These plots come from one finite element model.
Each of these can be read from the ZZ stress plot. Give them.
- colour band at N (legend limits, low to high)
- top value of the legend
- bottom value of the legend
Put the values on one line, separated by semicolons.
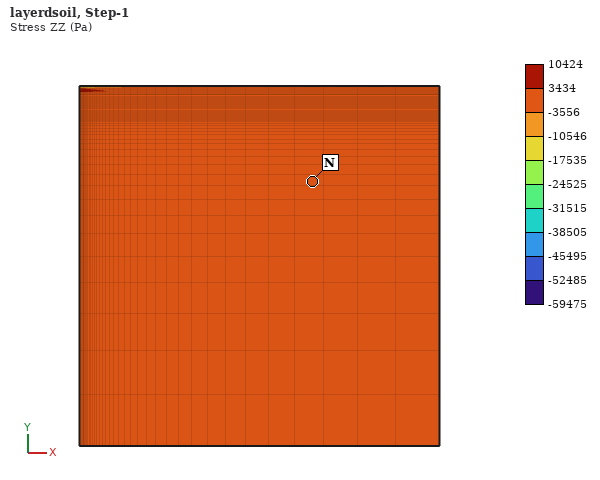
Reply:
-3556 to 3434 Pa; 10424 Pa; -59475 Pa
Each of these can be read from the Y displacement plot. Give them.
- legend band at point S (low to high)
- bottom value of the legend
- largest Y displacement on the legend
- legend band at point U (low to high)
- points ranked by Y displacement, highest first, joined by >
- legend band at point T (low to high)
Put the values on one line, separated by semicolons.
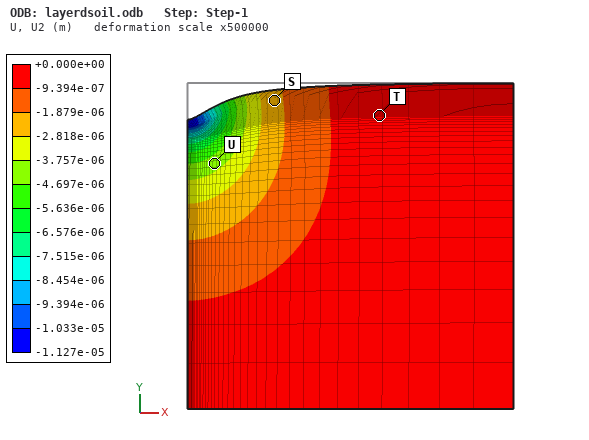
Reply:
-2.818e-06 to -1.879e-06 m; -1.127e-05 m; +0.000e+00 m; -4.697e-06 to -3.757e-06 m; T > S > U; -9.394e-07 to +0.000e+00 m
